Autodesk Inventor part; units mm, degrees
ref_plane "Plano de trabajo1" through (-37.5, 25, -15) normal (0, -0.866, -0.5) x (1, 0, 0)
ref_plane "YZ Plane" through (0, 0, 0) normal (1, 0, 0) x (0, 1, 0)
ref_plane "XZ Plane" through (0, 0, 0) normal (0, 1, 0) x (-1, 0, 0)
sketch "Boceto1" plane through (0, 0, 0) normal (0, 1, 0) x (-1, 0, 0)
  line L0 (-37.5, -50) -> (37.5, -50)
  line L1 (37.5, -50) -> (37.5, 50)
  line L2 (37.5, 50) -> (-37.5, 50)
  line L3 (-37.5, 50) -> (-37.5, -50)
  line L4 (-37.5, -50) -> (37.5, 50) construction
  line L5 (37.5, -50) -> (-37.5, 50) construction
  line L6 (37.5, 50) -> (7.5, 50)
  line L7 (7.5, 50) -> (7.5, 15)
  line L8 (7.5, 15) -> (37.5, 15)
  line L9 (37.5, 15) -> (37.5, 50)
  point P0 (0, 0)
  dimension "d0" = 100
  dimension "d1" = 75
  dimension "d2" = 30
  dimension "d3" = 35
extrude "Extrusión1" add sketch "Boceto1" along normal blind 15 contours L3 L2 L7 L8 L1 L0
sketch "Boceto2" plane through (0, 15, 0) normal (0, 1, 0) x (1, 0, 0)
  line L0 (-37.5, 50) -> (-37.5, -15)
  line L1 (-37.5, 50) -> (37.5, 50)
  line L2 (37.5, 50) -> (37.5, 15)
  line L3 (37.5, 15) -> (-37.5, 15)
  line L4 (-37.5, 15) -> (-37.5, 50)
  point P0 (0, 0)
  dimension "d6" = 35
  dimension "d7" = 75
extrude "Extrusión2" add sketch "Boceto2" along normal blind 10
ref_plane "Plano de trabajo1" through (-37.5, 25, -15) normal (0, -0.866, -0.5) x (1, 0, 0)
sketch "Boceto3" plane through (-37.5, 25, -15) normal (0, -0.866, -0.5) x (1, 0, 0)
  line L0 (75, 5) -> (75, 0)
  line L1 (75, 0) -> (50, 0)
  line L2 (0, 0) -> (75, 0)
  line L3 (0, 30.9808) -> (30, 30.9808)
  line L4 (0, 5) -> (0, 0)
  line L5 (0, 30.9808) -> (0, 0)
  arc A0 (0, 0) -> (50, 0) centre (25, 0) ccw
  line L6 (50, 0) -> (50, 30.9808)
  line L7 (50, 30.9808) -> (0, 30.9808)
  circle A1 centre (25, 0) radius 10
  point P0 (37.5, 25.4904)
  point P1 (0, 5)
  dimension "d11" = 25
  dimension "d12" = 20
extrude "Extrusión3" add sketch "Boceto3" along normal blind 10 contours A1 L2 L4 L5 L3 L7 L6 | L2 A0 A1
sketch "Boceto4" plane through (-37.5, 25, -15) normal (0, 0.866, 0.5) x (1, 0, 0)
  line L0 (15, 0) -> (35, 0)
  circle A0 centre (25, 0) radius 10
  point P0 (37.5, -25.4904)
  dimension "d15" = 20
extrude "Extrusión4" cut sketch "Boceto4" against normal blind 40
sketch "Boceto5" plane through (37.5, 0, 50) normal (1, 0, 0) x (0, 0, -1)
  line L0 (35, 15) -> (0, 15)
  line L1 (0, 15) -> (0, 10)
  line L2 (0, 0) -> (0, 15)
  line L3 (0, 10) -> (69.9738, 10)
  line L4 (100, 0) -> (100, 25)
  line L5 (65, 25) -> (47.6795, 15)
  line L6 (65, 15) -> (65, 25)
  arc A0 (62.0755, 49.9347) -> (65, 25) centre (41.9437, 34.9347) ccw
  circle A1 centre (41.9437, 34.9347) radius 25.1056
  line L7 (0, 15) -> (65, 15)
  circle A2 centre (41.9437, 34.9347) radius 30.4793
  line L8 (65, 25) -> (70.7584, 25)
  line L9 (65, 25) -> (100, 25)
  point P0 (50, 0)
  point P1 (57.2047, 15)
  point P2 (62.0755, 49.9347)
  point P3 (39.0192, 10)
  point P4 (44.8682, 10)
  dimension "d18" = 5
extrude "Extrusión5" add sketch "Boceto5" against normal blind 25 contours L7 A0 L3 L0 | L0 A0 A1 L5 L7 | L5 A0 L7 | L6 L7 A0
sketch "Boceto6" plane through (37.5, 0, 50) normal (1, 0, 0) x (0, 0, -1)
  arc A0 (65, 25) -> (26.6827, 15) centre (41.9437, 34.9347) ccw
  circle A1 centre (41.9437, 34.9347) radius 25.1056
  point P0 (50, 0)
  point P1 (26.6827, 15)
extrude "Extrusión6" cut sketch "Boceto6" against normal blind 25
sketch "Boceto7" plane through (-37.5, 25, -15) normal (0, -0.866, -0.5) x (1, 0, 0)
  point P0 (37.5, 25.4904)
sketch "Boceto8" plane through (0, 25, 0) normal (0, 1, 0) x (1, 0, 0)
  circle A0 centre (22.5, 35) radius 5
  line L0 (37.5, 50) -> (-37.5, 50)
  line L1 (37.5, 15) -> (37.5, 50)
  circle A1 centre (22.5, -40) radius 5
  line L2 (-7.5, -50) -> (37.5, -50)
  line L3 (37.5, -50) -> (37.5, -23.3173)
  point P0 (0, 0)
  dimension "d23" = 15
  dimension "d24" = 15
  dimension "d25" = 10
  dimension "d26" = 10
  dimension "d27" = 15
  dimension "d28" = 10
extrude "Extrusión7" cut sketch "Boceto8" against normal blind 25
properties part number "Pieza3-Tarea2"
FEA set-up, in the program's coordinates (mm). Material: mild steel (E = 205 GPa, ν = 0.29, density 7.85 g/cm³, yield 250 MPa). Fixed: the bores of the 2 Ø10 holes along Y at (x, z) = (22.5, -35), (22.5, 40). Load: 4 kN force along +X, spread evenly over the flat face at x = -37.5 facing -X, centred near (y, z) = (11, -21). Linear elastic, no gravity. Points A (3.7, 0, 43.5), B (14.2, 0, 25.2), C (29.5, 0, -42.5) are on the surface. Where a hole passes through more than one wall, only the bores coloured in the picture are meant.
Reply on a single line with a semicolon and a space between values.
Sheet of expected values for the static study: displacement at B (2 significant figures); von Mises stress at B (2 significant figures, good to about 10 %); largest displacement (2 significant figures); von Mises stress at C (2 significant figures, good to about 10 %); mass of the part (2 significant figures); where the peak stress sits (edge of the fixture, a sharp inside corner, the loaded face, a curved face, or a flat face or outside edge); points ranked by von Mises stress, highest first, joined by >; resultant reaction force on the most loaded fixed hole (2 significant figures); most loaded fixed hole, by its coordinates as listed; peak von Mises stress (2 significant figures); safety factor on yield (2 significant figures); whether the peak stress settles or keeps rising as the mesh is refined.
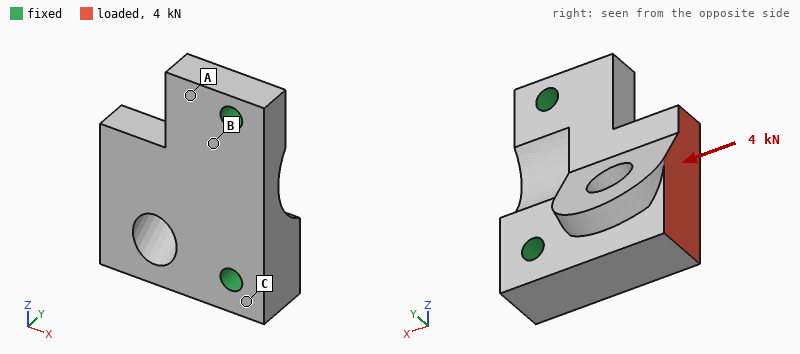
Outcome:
0.40 µm; 3.6 MPa; 1.8 µm; 2.0 MPa; 930 g; a curved face; B > C > A; 3.3 kN; (22.5, -35); 13 MPa; 20; settles
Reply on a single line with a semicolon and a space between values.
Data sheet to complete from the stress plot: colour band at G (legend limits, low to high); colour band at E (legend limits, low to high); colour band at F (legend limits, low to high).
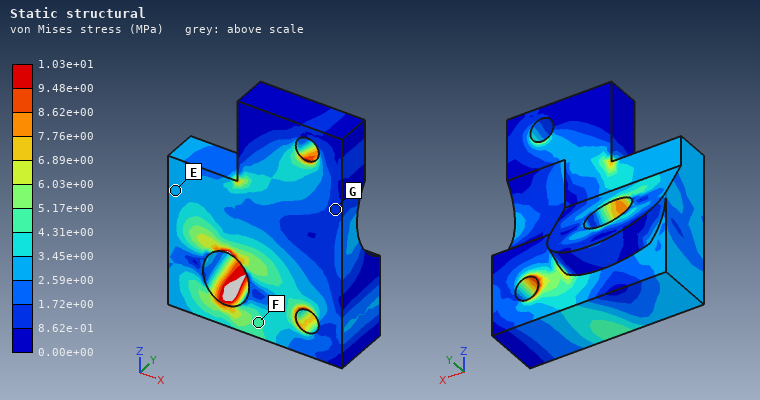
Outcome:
8.62e-01 to 1.72e+00 MPa; 2.59e+00 to 3.45e+00 MPa; 4.31e+00 to 5.17e+00 MPa
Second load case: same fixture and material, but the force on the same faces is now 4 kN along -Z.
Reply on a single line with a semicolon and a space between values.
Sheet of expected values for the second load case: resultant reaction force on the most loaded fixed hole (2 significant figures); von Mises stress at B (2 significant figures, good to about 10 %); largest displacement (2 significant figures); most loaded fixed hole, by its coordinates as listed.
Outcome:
3.7 kN; 11 MPa; 8.7 µm; (22.5, 40)
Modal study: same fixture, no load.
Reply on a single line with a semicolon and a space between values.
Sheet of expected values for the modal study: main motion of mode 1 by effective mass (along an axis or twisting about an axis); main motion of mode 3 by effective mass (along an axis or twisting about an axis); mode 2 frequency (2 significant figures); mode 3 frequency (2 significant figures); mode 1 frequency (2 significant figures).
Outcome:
along Y; along Z; 7700 Hz; 8700 Hz; 4100 Hz
